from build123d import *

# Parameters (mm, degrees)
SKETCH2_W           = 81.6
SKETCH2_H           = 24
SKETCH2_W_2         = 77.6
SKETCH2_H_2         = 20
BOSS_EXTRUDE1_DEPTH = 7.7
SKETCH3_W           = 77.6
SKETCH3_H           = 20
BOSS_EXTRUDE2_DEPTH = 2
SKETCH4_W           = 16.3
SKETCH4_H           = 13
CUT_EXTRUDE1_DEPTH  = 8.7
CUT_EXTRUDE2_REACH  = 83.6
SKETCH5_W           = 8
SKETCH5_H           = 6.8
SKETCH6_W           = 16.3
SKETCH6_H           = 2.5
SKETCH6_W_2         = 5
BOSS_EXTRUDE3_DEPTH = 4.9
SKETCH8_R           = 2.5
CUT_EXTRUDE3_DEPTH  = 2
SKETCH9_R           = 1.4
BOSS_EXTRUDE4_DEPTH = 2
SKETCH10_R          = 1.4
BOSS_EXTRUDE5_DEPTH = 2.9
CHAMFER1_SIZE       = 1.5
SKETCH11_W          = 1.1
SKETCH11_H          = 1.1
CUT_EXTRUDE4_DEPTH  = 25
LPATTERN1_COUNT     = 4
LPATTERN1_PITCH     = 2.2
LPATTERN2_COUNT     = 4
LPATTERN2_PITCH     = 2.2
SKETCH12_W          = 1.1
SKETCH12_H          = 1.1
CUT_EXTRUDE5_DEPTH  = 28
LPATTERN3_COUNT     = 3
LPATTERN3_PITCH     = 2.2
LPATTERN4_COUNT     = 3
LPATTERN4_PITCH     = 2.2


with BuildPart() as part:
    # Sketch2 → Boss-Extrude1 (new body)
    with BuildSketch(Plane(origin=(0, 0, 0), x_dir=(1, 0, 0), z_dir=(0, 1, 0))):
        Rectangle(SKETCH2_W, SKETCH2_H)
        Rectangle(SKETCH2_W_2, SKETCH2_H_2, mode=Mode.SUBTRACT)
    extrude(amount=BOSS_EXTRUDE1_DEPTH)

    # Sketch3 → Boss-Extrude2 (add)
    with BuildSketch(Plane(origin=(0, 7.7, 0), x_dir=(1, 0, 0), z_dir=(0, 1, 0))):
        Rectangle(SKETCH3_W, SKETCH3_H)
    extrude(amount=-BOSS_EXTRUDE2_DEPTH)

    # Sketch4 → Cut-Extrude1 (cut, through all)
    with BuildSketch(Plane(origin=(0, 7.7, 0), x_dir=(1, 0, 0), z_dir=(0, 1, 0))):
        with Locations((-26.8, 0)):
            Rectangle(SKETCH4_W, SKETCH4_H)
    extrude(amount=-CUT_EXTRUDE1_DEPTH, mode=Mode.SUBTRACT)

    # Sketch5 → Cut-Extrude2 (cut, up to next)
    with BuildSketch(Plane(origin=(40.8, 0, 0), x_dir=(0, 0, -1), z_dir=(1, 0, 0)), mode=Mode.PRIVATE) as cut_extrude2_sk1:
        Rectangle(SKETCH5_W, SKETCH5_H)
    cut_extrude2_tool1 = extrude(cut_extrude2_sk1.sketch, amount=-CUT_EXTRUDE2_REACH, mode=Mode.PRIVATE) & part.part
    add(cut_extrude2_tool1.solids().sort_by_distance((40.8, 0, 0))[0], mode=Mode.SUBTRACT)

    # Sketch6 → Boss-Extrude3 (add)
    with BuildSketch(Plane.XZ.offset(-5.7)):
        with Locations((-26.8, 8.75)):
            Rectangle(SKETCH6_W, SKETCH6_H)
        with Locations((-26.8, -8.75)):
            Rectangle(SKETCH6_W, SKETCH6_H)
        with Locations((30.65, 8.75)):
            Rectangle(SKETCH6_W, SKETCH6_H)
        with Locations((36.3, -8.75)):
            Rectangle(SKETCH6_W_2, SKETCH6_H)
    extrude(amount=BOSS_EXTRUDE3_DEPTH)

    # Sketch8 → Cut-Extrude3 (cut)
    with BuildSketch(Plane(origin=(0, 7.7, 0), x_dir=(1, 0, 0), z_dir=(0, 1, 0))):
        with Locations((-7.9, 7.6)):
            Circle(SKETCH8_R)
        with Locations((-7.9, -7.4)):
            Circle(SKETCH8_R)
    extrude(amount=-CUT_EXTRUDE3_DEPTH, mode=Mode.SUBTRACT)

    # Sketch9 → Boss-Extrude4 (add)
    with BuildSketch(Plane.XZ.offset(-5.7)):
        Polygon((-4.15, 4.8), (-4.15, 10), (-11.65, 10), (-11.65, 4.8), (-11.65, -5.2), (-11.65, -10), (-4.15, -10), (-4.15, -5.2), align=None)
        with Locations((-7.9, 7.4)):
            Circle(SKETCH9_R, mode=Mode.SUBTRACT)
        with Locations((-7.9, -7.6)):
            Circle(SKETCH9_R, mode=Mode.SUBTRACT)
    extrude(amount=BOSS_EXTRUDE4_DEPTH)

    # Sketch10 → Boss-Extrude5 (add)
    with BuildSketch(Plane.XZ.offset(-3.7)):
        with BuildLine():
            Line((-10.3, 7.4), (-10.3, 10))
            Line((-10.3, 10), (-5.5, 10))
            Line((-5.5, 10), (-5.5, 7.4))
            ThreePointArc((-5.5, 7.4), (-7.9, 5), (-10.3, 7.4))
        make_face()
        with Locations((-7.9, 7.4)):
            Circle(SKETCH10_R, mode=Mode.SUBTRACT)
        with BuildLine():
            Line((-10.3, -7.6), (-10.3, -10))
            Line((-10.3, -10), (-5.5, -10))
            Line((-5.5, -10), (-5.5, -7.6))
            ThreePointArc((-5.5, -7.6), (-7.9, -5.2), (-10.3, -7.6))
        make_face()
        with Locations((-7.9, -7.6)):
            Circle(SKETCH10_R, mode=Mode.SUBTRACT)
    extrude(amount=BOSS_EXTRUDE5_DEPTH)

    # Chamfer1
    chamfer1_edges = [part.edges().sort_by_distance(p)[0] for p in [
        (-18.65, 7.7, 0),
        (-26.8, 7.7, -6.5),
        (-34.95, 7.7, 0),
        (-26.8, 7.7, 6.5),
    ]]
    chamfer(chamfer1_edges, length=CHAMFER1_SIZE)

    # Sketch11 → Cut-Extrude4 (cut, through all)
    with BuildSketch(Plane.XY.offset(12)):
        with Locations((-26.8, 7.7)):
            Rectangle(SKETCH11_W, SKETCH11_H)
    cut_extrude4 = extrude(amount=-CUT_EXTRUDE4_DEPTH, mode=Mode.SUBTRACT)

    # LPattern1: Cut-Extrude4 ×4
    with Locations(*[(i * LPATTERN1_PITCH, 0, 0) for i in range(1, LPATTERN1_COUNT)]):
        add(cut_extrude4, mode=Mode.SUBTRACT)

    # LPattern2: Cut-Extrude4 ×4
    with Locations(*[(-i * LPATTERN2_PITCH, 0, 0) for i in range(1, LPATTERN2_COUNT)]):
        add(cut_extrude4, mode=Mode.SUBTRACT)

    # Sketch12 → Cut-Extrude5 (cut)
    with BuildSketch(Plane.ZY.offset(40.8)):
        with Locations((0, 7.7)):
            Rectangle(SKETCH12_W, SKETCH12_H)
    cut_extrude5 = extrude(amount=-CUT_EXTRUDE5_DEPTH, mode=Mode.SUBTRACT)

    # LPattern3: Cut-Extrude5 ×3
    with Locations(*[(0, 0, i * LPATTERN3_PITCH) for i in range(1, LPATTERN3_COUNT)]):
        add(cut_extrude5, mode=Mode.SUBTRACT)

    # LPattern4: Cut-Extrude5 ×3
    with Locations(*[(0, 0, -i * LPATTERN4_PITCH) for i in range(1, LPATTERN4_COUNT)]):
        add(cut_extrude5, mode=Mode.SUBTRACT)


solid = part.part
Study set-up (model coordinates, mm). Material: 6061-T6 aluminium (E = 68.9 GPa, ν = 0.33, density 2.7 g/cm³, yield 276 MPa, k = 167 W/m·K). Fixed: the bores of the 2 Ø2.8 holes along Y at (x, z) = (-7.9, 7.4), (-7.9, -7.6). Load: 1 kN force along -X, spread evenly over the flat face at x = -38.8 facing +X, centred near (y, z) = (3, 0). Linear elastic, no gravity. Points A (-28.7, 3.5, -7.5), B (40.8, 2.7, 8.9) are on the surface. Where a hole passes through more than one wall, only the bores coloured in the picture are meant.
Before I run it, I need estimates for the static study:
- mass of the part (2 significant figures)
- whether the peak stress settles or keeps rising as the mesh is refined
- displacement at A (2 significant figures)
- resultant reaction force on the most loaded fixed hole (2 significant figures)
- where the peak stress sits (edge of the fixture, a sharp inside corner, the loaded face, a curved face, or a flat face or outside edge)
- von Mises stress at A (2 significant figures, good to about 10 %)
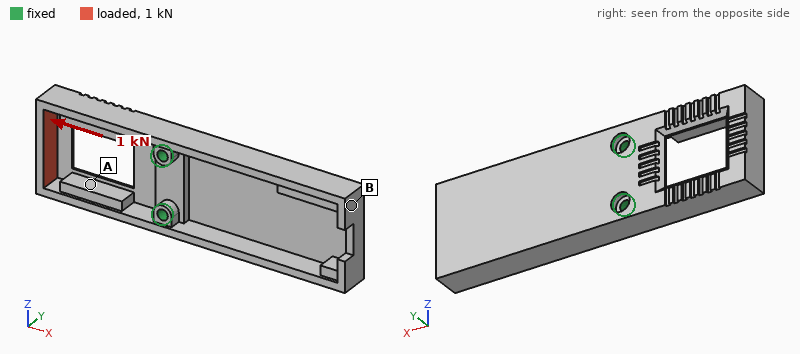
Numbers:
18 g
keeps rising
0.029 mm
500 N
a sharp inside corner
26 MPa
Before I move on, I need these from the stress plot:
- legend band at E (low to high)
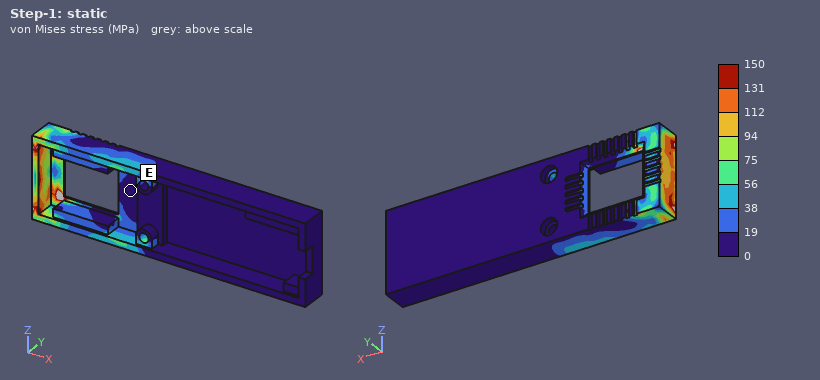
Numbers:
0 to 19 MPa
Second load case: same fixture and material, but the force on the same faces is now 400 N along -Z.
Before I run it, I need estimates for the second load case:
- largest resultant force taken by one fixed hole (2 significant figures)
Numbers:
710 N
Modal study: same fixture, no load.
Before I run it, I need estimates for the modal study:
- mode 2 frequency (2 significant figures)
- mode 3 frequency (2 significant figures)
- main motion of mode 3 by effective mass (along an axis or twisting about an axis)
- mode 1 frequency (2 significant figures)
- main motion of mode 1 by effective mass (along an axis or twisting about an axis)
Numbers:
3000 Hz
3600 Hz
along Y
1700 Hz
along Y
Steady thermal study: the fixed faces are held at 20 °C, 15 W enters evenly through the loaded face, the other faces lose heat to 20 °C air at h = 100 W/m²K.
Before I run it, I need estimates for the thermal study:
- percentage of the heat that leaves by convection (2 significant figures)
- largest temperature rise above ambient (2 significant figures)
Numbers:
34 %
48 K
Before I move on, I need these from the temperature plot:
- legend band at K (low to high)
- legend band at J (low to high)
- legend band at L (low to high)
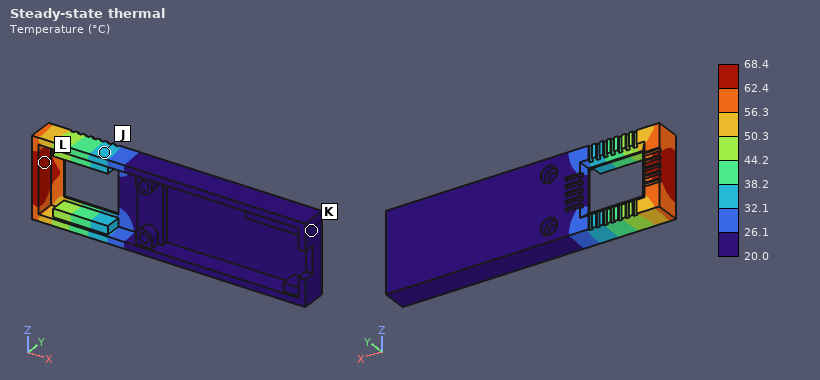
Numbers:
20.0 to 26.1 °C
32.1 to 38.2 °C
62.4 to 68.4 °C
